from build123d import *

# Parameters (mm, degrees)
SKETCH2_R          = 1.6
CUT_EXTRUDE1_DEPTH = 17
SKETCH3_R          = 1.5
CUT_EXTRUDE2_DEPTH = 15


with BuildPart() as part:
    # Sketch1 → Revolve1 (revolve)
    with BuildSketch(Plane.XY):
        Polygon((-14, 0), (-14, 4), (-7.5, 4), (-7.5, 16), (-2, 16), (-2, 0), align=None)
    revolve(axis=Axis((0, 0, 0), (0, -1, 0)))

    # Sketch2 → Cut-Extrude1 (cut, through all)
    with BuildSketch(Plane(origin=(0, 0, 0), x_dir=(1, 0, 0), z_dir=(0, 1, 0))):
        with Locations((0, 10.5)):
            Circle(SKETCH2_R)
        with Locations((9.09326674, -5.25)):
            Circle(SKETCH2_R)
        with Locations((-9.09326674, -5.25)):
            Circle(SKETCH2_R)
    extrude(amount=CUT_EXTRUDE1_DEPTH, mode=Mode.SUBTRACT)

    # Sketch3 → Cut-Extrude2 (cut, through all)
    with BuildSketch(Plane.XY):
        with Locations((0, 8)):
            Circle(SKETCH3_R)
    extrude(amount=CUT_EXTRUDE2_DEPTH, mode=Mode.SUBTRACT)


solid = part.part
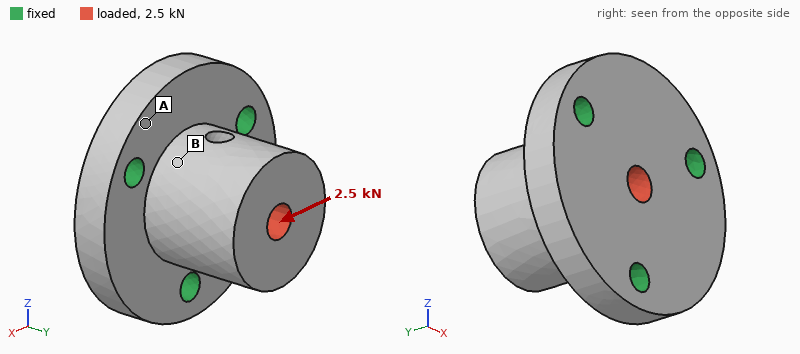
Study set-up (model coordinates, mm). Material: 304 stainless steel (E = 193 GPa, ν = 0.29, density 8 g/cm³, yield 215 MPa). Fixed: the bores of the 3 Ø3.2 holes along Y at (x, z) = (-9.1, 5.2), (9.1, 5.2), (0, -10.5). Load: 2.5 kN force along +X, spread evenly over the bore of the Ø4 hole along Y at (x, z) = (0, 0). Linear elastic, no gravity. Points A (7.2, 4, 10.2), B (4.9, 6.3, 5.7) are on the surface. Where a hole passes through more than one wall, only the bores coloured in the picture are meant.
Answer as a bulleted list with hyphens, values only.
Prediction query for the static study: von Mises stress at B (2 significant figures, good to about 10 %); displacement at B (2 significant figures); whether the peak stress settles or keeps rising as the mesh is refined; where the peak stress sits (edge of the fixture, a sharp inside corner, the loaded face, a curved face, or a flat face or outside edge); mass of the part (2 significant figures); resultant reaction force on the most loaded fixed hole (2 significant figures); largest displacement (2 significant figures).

- 35 MPa
- 2.4 µm
- keeps rising
- edge of the fixture
- 34 g
- 1.3 kN
- 6.9 µm
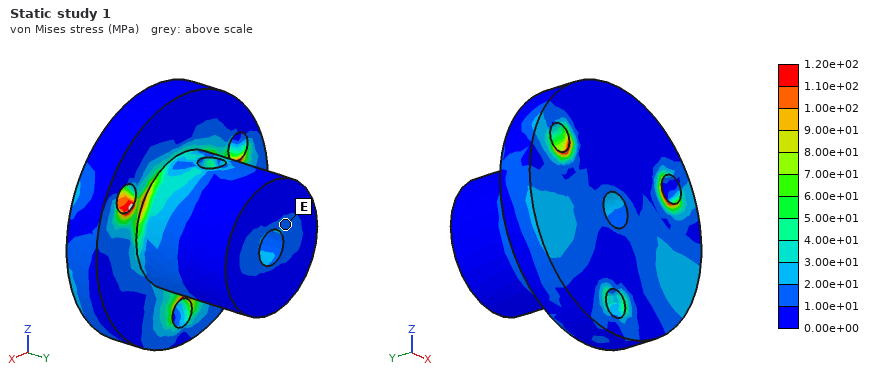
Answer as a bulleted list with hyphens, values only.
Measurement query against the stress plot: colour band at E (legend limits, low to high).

- 1.00e+01 to 2.00e+01 MPa
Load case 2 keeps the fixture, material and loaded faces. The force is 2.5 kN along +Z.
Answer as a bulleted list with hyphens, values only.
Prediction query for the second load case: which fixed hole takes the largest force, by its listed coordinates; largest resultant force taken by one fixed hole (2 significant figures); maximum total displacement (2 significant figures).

- (0, -10.5)
- 1.4 kN
- 6.8 µm
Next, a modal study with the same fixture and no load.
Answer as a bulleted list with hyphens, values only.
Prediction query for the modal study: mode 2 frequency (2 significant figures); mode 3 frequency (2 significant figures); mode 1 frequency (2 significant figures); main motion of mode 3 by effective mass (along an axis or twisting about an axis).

- 24 kHz
- 34 kHz
- 24 kHz
- along Y
